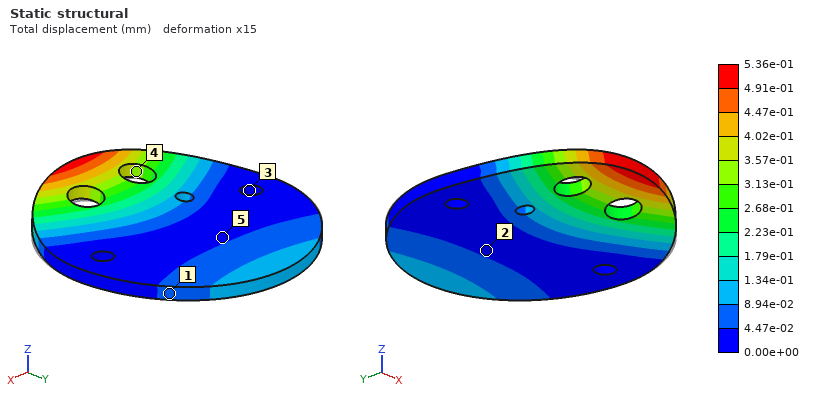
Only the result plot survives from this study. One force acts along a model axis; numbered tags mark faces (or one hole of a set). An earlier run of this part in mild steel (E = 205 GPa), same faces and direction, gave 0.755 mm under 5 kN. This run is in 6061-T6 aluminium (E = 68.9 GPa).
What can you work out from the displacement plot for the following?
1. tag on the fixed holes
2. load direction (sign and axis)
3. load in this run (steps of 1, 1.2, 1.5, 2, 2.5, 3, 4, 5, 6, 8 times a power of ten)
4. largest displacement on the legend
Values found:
3
+Z
1.2 kN
5.36e-01 mm
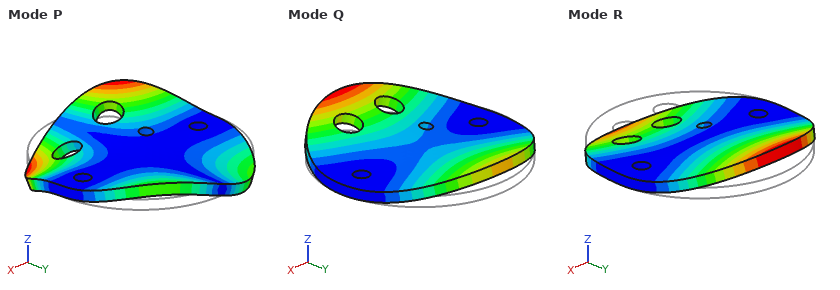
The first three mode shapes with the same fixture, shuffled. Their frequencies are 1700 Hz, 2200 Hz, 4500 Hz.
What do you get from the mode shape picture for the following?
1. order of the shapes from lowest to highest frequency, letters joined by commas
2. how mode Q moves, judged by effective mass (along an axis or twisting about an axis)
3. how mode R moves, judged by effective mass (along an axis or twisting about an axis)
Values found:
R, Q, P
along Z
twisting about X
